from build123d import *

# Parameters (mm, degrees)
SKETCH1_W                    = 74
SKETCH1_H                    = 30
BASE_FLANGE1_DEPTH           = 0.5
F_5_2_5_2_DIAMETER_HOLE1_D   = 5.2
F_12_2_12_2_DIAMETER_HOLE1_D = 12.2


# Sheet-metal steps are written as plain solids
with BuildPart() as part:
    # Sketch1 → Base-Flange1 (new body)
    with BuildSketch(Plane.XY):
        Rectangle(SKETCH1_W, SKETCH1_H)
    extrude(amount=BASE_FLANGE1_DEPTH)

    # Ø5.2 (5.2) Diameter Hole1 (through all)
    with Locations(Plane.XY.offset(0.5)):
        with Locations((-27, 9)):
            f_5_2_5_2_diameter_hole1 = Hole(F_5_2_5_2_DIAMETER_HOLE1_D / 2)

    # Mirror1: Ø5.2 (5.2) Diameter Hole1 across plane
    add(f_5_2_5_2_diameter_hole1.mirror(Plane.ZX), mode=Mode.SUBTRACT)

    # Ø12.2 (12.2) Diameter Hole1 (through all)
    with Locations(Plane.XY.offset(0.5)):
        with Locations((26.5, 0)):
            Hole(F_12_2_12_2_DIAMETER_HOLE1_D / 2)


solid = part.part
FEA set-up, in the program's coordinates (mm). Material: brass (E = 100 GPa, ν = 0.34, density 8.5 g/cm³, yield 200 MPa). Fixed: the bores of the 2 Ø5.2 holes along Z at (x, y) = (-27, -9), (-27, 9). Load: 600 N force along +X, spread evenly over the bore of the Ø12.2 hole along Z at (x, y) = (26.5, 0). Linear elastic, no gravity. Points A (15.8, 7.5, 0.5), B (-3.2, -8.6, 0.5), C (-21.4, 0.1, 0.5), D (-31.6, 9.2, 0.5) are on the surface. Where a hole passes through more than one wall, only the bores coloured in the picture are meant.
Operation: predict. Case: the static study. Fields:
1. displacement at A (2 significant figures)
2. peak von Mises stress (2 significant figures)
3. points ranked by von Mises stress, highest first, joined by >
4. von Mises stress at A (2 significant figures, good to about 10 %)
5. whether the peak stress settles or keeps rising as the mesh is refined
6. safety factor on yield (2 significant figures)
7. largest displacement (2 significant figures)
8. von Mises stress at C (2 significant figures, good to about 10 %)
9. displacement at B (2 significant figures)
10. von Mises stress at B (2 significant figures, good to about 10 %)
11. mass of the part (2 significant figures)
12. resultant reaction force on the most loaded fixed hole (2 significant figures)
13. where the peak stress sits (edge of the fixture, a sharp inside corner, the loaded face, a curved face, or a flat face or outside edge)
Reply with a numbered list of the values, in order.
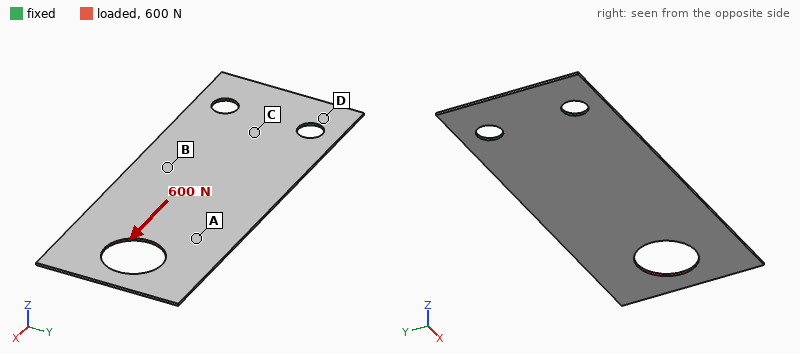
1. 17 µm
2. 130 MPa
3. A > B > C > D
4. 50 MPa
5. settles
6. 1.5
7. 36 µm
8. 24 MPa
9. 9.6 µm
10. 40 MPa
11. 8.8 g
12. 300 N
13. the loaded face
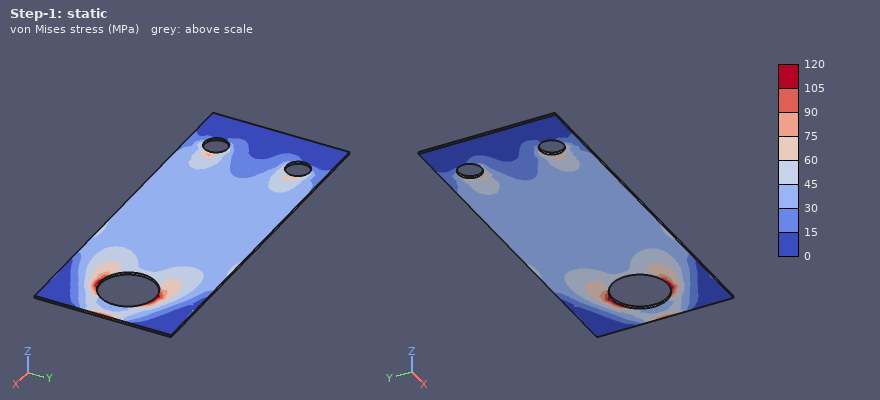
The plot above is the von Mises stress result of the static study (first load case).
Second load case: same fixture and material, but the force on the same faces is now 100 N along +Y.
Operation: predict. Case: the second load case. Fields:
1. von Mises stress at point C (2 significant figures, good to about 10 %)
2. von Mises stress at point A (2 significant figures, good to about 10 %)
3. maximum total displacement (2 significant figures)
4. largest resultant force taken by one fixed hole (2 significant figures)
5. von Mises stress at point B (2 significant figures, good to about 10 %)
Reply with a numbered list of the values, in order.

1. 14 MPa
2. 10 MPa
3. 77 µm
4. 260 N
5. 25 MPa
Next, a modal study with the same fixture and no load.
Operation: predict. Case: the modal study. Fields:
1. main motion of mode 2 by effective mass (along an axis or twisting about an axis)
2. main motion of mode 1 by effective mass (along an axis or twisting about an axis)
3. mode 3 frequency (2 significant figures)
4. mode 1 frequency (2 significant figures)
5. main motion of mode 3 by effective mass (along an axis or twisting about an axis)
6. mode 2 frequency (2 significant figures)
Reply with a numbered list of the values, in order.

1. twisting about X
2. along Z
3. 450 Hz
4. 80 Hz
5. along Z
6. 320 Hz
